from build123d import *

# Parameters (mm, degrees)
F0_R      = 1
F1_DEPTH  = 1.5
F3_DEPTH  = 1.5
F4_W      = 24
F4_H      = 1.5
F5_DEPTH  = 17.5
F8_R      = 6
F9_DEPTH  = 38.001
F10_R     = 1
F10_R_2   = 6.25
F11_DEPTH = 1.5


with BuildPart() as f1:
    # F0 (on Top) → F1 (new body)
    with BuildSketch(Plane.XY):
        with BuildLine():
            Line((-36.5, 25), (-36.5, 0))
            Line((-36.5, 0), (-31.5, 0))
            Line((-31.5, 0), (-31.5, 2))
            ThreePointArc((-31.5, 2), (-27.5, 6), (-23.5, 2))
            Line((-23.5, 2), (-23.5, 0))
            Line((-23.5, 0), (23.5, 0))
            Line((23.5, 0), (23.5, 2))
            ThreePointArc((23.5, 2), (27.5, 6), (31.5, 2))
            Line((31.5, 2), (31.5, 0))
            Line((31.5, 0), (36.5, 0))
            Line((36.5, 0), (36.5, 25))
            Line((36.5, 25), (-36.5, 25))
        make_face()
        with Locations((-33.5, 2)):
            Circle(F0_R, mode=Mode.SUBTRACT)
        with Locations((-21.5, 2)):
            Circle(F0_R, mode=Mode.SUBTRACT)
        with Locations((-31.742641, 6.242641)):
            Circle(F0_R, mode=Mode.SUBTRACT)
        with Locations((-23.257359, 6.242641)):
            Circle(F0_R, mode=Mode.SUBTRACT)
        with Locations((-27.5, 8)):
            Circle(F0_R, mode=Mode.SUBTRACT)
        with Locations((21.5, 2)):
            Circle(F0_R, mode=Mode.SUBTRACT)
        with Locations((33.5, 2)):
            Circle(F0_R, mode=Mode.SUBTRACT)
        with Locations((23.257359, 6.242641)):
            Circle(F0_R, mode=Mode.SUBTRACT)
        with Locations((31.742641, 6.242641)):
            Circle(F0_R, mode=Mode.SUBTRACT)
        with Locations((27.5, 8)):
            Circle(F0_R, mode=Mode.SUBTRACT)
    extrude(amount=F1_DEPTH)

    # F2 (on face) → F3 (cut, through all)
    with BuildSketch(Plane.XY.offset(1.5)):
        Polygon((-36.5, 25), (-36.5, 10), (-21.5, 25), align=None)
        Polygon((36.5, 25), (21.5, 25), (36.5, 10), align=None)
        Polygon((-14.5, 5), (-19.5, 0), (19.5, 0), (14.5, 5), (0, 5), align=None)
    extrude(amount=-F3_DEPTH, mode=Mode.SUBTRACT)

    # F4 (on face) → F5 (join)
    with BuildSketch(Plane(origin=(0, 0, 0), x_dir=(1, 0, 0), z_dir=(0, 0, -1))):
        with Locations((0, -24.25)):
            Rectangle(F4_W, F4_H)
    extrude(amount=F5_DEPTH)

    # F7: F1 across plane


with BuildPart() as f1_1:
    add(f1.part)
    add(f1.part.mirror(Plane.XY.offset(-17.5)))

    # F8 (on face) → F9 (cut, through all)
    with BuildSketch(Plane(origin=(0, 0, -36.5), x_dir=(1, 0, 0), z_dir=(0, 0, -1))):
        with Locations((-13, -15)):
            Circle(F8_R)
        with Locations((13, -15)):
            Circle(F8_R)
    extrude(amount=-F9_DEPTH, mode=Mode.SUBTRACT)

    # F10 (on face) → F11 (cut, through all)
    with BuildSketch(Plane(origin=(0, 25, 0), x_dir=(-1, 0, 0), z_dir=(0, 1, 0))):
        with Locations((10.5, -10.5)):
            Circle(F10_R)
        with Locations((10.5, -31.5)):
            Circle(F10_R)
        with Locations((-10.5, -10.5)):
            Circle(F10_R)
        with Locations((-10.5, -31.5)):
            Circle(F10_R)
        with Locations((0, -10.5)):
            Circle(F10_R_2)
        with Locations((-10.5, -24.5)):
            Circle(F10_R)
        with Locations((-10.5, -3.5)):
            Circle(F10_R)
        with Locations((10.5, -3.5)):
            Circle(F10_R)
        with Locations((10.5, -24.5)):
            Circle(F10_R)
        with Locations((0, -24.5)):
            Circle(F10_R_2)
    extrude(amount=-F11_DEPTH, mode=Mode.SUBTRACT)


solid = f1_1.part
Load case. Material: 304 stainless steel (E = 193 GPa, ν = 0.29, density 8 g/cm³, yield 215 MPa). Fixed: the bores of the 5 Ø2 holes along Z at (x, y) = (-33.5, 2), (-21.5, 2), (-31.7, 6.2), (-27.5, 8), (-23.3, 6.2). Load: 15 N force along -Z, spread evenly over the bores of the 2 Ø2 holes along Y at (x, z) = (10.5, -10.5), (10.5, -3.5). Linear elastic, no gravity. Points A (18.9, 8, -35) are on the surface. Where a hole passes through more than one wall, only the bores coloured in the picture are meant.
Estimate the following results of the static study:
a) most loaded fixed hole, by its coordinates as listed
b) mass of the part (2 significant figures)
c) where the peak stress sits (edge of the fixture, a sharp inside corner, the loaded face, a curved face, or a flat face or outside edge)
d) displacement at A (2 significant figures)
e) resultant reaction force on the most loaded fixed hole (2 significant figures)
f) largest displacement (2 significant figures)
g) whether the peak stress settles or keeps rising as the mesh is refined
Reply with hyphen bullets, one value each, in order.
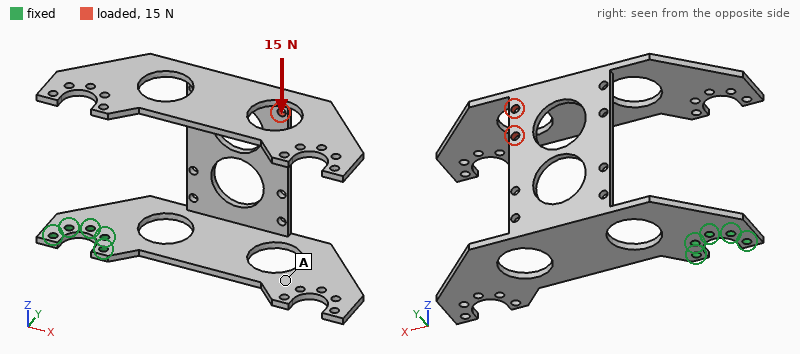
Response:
- (-23.3, 6.2)
- 33 g
- edge of the fixture
- 0.36 mm
- 56 N
- 0.78 mm
- keeps rising
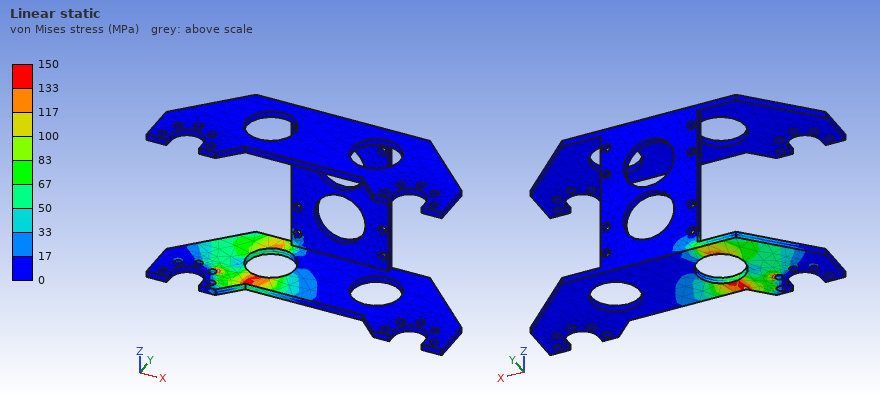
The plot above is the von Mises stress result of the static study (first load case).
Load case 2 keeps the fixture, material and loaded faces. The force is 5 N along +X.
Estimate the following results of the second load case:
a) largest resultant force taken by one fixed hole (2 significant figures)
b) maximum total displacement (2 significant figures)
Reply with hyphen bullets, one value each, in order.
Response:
- 12 N
- 0.26 mm
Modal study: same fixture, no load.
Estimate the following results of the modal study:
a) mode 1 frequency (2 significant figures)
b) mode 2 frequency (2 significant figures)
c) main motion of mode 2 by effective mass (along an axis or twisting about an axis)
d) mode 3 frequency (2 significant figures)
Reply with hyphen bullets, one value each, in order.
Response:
- 140 Hz
- 180 Hz
- along Y
- 360 Hz
